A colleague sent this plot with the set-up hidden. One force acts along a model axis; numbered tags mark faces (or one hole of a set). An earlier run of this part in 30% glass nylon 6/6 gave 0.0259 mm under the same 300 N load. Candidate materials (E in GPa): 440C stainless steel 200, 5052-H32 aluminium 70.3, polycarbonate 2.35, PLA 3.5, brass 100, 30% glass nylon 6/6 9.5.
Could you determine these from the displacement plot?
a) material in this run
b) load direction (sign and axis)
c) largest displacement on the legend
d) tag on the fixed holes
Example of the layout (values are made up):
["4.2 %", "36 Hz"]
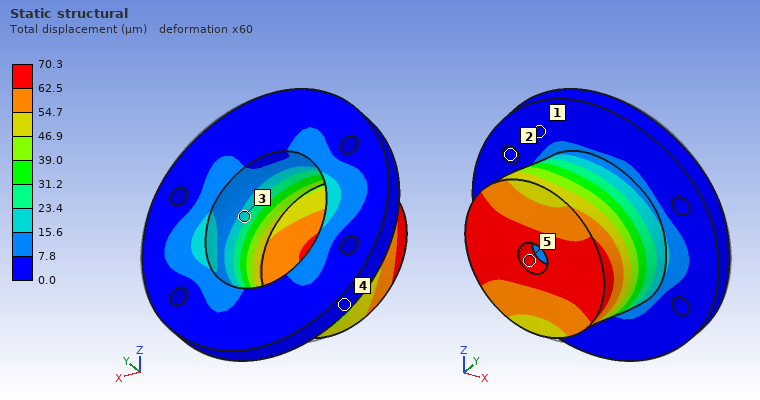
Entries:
["PLA", "-X", "70.3 µm", "2"]
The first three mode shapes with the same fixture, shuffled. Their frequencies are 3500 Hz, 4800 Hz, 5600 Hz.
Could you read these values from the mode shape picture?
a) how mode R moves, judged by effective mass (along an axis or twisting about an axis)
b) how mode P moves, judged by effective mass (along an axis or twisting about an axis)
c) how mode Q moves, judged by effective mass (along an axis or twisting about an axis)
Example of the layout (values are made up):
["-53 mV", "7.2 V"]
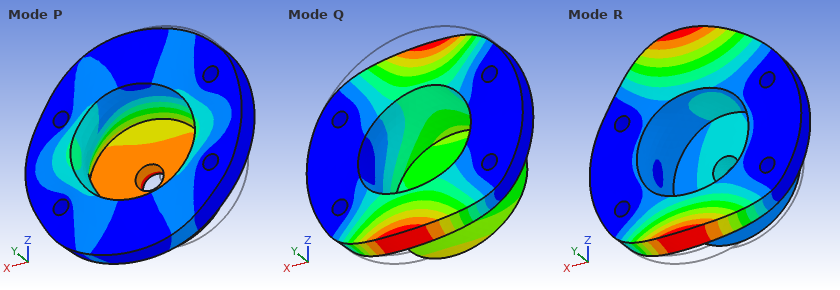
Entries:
["along Y", "along X", "along Z"]
